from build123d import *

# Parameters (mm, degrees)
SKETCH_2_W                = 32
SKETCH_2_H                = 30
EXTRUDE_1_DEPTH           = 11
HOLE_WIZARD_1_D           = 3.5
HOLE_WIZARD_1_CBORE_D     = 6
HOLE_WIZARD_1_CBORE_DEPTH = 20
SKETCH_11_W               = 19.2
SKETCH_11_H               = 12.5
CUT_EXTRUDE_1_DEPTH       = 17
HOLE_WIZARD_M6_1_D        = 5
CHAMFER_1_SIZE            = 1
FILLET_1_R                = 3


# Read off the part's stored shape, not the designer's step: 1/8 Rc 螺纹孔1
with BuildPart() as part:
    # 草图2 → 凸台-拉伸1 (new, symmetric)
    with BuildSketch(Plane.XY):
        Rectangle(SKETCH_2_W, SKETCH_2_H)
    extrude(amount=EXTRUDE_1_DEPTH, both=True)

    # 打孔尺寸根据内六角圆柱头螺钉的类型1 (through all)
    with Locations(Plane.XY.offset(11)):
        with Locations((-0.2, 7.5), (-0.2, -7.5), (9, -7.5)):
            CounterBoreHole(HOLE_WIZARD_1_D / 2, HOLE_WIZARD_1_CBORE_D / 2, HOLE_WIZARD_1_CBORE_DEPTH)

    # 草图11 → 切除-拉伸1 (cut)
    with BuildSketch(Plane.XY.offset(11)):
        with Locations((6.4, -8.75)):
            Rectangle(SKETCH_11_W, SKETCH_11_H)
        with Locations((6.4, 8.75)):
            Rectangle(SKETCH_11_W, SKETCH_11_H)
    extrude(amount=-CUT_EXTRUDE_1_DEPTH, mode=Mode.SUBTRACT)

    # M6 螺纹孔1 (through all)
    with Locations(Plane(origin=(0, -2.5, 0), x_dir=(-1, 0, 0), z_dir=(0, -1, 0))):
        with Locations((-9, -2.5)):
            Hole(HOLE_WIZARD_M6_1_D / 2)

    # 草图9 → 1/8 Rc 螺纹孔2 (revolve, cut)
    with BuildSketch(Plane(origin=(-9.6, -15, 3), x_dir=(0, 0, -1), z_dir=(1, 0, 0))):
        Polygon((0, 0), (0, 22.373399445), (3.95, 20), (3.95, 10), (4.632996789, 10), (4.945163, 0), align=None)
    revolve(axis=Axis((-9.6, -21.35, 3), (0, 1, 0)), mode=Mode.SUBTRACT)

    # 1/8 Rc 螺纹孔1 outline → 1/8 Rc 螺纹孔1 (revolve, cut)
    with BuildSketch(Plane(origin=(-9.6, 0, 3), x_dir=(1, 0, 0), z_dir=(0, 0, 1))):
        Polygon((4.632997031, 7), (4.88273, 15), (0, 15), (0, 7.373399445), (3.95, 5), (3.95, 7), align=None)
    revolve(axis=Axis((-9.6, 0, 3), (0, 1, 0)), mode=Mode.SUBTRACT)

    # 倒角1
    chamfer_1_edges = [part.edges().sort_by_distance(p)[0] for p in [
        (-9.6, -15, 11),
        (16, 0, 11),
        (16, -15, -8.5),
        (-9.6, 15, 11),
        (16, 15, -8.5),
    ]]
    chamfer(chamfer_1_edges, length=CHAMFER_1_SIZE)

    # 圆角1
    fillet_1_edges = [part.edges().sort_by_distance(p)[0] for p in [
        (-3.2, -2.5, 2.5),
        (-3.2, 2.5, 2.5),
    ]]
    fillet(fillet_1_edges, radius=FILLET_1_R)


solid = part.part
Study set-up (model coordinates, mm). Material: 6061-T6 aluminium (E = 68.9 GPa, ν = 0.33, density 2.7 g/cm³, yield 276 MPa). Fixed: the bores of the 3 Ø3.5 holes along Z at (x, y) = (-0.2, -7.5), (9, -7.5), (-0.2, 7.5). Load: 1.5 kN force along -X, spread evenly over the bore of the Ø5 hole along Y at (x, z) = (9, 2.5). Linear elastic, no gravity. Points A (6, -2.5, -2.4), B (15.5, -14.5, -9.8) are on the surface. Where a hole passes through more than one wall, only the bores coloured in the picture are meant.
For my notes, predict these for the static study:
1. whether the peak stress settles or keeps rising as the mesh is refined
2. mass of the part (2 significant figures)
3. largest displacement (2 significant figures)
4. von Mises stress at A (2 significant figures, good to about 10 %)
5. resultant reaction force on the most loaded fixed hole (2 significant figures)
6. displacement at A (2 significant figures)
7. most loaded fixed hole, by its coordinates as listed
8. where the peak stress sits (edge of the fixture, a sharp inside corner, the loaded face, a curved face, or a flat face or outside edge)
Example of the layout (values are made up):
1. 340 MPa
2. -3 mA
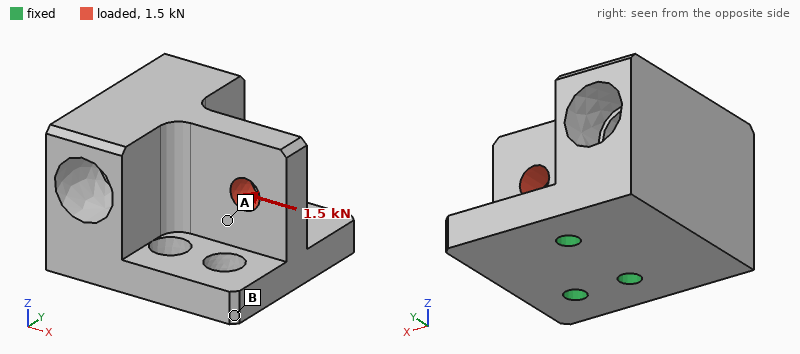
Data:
1. keeps rising
2. 29 g
3. 76 µm
4. 55 MPa
5. 1.6 kN
6. 26 µm
7. (9, -7.5)
8. edge of the fixture
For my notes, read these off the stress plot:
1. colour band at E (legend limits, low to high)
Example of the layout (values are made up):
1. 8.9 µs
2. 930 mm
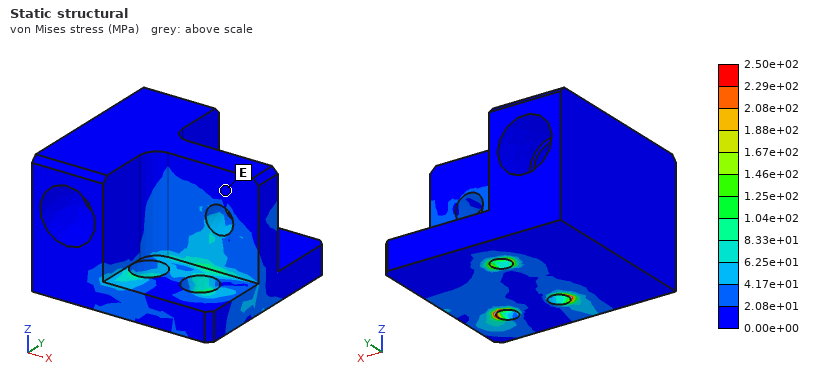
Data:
1. 0.00e+00 to 2.08e+01 MPa
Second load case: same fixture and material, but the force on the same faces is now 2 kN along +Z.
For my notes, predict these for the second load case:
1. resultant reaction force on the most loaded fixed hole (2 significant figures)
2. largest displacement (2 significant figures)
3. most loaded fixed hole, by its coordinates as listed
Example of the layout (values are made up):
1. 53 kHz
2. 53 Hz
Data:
1. 1.6 kN
2. 59 µm
3. (9, -7.5)
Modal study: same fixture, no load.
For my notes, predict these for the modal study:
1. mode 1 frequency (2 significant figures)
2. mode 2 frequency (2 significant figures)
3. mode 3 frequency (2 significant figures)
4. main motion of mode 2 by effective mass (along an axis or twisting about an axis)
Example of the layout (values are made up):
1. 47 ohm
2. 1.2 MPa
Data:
1. 5300 Hz
2. 9500 Hz
3. 16 kHz
4. along Y
